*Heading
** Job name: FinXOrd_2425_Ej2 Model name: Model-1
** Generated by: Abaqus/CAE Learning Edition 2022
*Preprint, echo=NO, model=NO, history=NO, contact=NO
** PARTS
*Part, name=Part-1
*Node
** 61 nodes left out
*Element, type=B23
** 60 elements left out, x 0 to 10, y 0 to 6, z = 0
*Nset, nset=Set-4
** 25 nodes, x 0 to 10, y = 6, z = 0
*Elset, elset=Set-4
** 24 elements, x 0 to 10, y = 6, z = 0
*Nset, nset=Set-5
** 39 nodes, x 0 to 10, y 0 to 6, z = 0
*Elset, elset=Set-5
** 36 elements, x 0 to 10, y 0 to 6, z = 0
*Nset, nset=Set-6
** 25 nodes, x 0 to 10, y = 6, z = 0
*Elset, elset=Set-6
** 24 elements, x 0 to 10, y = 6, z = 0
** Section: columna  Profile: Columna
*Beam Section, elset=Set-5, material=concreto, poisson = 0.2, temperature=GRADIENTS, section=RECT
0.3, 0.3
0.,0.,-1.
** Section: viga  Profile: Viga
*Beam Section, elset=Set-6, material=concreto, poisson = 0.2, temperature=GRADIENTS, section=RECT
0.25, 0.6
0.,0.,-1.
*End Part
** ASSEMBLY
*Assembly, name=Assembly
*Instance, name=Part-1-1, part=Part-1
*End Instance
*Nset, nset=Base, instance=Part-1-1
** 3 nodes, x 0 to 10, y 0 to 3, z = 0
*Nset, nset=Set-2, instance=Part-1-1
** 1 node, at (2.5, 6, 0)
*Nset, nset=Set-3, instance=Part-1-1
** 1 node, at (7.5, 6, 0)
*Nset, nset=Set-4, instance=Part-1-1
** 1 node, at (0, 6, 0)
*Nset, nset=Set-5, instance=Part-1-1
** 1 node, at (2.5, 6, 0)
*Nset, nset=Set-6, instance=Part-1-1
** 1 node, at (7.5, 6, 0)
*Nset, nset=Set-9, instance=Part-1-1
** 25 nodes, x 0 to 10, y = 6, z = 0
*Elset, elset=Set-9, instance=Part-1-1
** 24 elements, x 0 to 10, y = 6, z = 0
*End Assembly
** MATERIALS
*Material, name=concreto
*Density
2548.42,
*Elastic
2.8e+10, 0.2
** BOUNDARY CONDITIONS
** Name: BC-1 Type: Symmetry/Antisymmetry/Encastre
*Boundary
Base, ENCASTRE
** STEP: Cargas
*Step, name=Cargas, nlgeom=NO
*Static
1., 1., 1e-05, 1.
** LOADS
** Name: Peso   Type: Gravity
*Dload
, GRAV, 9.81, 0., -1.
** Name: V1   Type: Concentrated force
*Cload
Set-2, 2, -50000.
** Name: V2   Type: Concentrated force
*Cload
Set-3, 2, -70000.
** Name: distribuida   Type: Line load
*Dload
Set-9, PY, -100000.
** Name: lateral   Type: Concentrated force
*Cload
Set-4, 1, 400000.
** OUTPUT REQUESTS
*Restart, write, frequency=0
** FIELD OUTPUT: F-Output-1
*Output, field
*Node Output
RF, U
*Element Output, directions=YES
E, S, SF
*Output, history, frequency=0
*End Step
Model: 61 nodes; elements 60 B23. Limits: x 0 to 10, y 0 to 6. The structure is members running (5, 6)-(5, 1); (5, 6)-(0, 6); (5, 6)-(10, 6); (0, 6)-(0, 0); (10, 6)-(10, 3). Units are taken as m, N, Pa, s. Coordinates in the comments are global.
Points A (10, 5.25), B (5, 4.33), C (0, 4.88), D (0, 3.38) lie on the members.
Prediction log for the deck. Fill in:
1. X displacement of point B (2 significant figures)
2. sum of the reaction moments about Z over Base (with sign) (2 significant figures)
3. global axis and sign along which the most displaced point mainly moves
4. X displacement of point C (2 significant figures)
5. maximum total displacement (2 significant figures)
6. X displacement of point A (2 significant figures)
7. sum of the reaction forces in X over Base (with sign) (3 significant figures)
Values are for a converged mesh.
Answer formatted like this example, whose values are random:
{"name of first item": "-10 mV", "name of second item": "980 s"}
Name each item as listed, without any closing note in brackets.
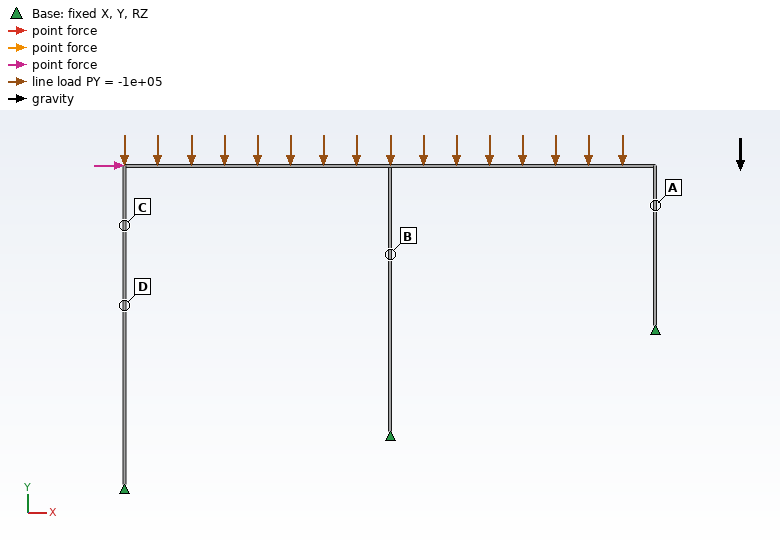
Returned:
{"X displacement of point B": "0.029 m", "sum of the reaction moments about Z over Base (with sign)": "7.4e+05 N·m", "global axis and sign along which the most displaced point mainly moves": "+X", "X displacement of point C": "0.033 m", "maximum total displacement": "0.039 m", "X displacement of point A": "0.031 m", "sum of the reaction forces in X over Base (with sign)": "-4.00e+05 N"}
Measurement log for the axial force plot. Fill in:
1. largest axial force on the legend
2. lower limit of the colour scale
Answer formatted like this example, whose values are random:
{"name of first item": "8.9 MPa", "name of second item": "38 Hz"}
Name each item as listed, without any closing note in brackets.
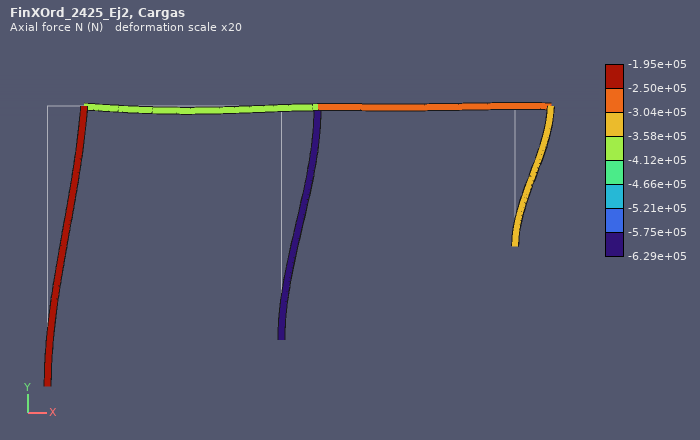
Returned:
{"largest axial force on the legend": "-1.95e+05 N", "lower limit of the colour scale": "-6.29e+05 N"}
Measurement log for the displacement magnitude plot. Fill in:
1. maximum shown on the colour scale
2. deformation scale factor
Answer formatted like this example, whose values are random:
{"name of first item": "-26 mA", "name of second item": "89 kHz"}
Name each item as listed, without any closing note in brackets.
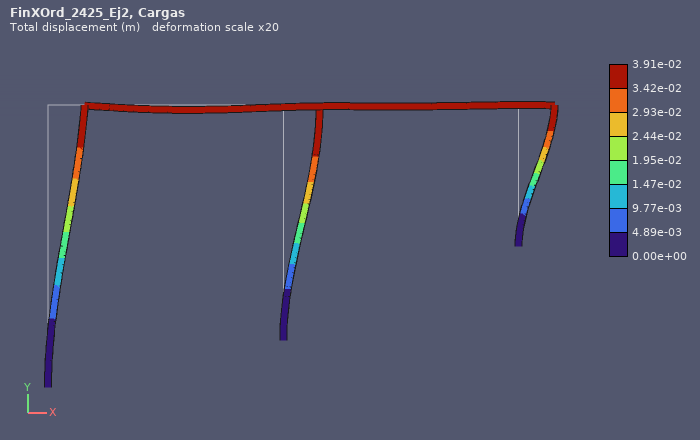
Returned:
{"maximum shown on the colour scale": "3.91e-02 m", "deformation scale factor": "20"}
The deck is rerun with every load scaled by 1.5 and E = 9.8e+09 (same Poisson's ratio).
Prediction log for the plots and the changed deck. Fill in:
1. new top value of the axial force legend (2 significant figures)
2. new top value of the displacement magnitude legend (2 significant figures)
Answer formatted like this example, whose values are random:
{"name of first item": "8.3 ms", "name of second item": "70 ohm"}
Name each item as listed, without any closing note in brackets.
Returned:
{"new top value of the axial force legend": "-2.9e+05 N", "new top value of the displacement magnitude legend": "0.17 m"}
